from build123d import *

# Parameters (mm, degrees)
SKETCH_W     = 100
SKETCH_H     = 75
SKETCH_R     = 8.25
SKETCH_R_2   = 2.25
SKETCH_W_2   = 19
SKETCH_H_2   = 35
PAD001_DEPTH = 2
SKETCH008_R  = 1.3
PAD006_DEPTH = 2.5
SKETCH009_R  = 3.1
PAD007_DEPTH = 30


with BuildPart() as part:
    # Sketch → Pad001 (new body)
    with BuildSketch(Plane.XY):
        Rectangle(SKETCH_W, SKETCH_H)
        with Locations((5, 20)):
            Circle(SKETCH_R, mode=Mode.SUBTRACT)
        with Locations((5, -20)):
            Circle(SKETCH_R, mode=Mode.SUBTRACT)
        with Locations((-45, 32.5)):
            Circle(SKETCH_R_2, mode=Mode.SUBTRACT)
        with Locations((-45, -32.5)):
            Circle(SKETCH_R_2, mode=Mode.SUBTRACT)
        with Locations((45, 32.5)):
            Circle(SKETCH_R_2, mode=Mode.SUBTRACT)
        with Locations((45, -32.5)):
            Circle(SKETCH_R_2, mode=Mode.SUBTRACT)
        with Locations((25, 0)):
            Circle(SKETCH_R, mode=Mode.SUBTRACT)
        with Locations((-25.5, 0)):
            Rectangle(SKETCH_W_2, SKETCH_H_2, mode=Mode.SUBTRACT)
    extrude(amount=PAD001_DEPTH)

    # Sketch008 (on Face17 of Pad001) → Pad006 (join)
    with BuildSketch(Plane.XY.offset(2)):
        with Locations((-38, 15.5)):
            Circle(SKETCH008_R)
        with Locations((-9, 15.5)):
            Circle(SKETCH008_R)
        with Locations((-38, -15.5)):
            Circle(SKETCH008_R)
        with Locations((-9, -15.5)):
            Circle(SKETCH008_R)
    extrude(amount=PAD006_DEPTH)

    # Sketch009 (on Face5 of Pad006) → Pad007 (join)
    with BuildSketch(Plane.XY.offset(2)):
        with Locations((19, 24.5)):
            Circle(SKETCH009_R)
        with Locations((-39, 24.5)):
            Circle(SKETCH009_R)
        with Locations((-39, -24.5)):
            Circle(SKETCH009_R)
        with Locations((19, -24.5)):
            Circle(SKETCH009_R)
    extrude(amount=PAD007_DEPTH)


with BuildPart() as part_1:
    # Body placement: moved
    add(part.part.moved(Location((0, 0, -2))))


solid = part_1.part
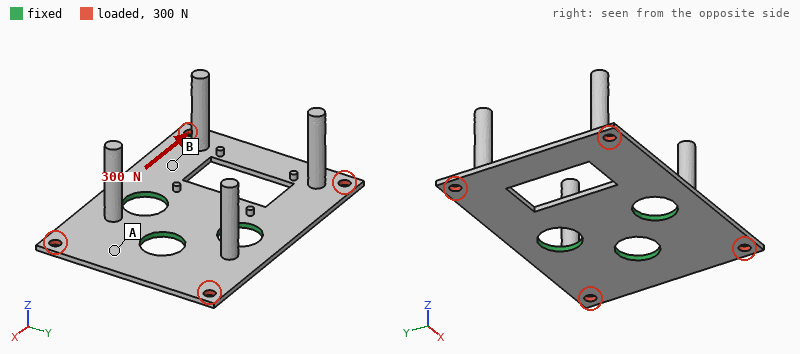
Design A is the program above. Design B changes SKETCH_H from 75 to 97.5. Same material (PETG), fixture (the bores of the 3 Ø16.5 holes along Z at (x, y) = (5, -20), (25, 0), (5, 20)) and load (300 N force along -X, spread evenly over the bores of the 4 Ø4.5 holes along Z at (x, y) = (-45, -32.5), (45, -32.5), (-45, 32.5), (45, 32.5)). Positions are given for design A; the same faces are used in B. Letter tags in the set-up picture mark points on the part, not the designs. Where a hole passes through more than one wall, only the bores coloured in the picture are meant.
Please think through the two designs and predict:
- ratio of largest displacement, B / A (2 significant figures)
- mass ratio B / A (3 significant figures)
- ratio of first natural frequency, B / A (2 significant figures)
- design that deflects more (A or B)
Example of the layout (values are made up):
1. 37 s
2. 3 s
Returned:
1. 0.81
2. 1.28
3. 1.1
4. A
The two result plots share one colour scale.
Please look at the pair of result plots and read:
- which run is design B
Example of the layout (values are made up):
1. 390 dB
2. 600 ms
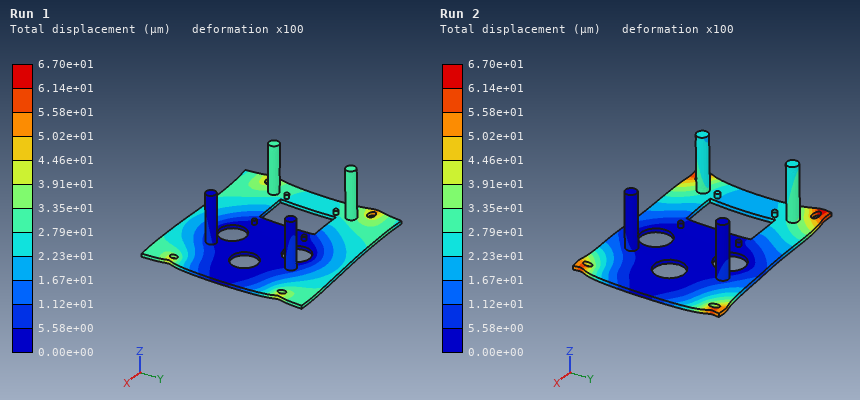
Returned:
1. Run 1
